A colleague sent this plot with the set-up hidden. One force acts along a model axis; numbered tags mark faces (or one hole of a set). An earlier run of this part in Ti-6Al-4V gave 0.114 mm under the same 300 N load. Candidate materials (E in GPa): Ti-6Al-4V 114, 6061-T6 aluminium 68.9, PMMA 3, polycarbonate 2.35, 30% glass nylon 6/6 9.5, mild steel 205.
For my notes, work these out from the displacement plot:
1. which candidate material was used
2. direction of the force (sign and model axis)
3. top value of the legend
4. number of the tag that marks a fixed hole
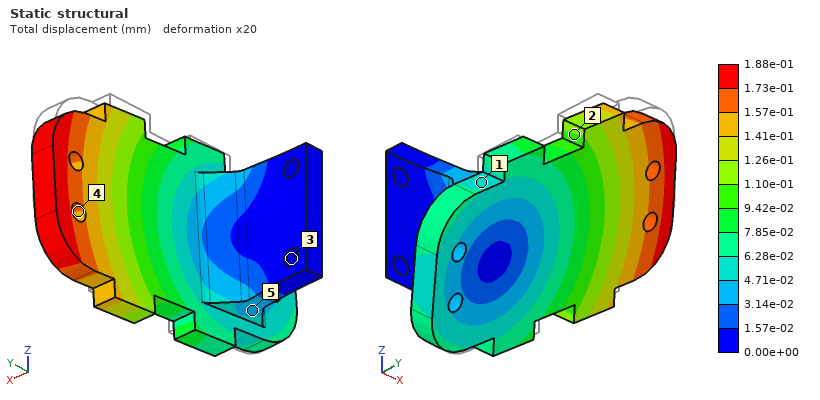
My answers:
6061-T6 aluminium
-Z
1.88e-01 mm
3
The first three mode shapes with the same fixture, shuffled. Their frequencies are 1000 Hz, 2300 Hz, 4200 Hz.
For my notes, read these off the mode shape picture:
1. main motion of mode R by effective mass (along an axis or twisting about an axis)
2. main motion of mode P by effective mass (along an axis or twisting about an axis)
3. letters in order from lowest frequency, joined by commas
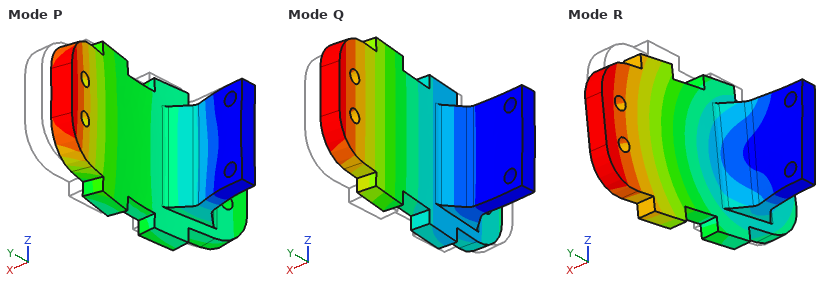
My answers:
along Z
along Y
Q, R, P
